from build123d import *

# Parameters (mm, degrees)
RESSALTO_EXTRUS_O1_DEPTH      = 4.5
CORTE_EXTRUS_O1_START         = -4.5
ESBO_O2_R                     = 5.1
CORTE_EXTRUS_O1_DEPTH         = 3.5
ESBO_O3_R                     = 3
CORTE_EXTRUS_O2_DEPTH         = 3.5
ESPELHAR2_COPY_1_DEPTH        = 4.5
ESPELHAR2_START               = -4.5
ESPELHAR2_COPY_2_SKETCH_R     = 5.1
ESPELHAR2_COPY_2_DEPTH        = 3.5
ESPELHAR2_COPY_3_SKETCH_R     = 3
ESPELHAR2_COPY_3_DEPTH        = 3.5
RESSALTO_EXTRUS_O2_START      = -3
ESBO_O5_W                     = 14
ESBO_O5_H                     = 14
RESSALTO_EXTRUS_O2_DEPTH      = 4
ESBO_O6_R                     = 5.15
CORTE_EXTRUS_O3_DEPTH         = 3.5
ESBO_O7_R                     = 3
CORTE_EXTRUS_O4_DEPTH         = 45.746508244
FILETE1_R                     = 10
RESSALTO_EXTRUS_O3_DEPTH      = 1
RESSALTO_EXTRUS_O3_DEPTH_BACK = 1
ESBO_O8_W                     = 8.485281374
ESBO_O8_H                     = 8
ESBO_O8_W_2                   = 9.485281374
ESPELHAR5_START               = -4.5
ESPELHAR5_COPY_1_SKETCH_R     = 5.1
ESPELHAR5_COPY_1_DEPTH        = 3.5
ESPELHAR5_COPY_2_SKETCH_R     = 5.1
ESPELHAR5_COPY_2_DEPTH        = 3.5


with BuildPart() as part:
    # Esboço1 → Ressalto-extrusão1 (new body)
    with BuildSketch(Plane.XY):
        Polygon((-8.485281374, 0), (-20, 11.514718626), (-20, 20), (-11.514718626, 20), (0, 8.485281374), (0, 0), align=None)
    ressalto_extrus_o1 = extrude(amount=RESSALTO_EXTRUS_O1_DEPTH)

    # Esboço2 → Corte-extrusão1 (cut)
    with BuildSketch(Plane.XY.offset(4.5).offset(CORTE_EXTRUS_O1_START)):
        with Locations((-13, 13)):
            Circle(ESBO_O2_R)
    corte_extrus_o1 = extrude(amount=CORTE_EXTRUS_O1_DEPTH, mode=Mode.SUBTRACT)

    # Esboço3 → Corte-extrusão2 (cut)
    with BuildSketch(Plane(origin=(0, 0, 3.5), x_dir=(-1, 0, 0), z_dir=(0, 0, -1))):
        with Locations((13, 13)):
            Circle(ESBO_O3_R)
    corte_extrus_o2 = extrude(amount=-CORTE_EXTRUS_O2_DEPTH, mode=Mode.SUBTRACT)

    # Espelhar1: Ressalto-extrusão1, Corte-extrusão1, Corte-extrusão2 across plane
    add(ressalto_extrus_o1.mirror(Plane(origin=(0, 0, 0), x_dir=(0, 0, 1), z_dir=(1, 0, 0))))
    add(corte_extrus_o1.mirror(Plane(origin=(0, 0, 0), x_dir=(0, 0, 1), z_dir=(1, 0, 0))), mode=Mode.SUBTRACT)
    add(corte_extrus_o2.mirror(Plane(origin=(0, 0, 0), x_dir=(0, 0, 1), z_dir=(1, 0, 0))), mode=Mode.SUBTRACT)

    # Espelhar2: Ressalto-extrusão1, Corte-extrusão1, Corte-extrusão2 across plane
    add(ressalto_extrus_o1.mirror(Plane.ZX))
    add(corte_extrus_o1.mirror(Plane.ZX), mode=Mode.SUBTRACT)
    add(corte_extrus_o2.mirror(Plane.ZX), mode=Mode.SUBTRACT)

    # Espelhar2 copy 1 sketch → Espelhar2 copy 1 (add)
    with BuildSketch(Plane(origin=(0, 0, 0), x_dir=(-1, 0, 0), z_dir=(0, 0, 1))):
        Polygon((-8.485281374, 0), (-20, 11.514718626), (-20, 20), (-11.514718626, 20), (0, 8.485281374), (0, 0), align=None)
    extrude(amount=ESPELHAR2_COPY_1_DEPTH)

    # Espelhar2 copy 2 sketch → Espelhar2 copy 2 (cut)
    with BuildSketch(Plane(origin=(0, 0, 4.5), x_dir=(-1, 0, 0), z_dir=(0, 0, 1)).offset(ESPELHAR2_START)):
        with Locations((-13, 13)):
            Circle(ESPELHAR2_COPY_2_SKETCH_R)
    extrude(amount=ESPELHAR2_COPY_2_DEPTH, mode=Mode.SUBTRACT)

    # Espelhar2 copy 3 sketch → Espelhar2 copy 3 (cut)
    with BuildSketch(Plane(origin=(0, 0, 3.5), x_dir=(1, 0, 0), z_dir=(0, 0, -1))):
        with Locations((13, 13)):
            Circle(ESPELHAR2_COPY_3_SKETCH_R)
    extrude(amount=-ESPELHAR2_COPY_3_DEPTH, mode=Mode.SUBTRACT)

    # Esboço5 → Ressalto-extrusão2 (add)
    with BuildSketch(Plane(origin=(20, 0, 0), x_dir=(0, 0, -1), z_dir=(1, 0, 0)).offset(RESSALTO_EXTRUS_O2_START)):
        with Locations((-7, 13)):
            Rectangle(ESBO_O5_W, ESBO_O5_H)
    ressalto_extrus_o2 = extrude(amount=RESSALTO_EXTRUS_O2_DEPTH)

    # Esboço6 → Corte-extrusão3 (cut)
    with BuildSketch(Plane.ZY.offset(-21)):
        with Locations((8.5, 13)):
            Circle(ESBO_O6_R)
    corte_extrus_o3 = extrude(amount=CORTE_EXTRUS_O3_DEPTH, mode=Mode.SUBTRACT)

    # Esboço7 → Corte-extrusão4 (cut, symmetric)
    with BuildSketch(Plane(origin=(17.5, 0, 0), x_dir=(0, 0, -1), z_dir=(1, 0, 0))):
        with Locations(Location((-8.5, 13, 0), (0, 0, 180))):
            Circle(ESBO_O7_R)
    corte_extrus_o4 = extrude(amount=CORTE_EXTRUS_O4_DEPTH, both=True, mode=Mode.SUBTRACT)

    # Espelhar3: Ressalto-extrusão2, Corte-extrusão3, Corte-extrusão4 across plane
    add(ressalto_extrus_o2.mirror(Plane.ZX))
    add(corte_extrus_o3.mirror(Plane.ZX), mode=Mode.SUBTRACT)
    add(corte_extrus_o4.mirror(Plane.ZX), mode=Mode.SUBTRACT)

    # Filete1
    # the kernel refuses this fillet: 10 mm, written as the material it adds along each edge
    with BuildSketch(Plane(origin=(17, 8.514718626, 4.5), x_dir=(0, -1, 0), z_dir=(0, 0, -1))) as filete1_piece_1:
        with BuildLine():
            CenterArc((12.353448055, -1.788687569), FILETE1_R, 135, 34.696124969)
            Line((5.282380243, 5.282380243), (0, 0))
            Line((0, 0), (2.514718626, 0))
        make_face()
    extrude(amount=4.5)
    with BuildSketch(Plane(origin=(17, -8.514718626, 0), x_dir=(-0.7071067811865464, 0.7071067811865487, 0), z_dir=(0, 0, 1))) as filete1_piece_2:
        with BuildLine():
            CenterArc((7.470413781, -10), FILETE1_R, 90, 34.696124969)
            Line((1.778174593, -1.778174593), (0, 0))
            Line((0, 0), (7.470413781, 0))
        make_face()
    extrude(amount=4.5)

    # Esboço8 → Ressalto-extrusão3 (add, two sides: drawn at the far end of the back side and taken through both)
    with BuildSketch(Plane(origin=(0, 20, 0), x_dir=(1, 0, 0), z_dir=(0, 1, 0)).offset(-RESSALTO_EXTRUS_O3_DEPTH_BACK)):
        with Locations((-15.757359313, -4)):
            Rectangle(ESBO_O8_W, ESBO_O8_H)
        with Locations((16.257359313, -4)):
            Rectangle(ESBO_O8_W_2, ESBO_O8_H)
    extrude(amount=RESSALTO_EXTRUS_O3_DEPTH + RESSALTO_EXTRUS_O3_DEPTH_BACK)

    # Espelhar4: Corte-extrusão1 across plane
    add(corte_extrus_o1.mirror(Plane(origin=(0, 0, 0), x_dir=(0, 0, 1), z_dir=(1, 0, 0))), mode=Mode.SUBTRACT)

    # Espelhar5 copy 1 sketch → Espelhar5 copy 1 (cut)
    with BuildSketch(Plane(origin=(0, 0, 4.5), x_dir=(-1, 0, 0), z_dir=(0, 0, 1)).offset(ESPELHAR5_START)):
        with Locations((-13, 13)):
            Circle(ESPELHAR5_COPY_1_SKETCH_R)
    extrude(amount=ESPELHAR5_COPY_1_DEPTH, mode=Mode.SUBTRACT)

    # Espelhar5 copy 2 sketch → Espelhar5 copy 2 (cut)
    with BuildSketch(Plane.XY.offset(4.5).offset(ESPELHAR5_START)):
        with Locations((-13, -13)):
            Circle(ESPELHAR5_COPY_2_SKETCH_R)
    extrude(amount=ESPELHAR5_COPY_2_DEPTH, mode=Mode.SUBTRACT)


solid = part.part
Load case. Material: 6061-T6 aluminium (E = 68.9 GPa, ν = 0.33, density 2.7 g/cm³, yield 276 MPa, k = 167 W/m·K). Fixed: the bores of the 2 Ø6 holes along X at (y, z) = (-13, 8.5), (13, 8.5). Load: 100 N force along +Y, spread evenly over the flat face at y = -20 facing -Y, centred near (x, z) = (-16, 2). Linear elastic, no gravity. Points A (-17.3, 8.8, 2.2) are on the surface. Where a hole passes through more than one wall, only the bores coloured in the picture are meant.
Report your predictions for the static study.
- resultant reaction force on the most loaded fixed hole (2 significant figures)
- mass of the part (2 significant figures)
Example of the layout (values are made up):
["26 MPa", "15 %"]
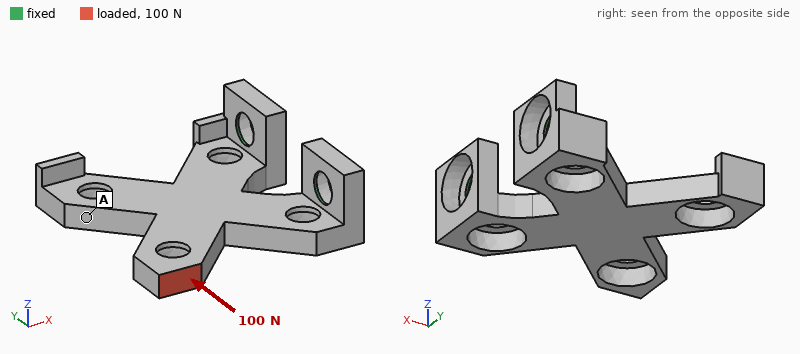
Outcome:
["130 N", "12 g"]
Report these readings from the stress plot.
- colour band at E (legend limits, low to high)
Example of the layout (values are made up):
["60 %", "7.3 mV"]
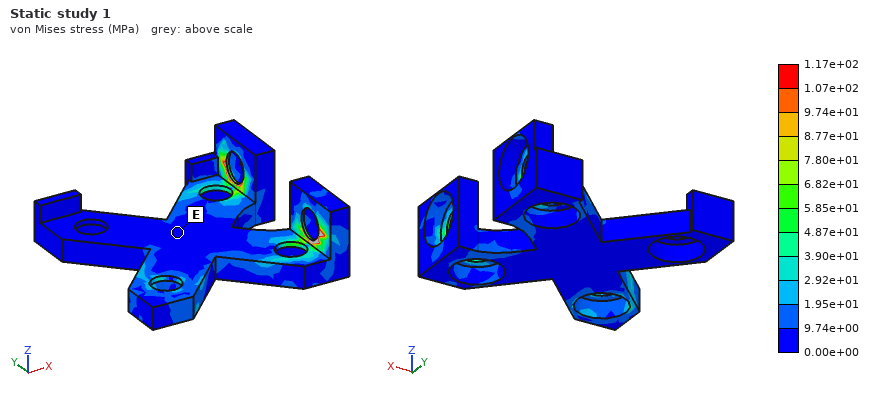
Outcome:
["0.00e+00 to 9.74e+00 MPa"]
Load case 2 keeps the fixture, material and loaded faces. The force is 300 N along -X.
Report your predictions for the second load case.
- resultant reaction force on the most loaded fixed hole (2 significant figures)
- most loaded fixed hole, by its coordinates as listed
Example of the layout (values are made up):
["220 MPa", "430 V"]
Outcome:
["370 N", "(-13, 8.5)"]
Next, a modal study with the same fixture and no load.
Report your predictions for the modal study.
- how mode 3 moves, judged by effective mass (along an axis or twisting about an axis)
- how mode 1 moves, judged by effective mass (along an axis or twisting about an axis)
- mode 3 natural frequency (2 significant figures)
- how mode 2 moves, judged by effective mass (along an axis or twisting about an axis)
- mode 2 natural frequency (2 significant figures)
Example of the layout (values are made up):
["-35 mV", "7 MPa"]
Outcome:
["along Y", "along Z", "4500 Hz", "along Y", "3300 Hz"]
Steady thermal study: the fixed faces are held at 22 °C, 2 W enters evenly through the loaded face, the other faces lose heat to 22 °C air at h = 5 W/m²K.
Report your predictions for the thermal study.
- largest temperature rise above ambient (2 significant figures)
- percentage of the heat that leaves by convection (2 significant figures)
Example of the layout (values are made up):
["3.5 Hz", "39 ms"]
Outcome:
["16 K", "4.5 %"]
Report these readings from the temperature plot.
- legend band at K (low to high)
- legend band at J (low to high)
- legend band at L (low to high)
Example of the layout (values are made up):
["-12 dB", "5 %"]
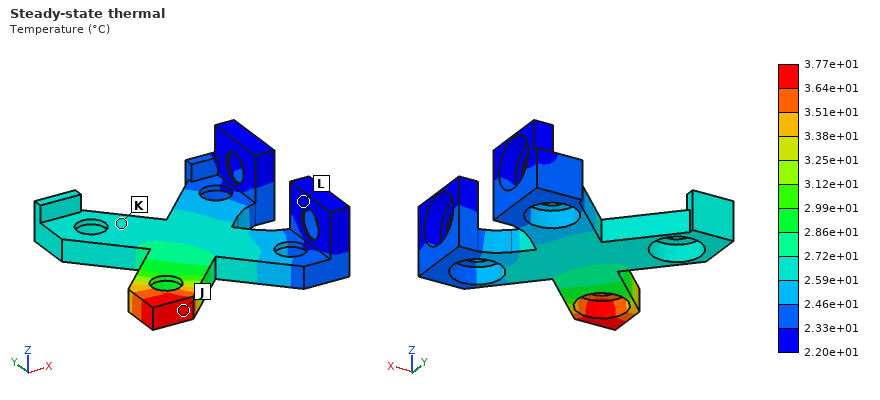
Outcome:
["2.59e+01 to 2.72e+01 °C", "3.64e+01 to 3.77e+01 °C", "2.20e+01 to 2.33e+01 °C"]
